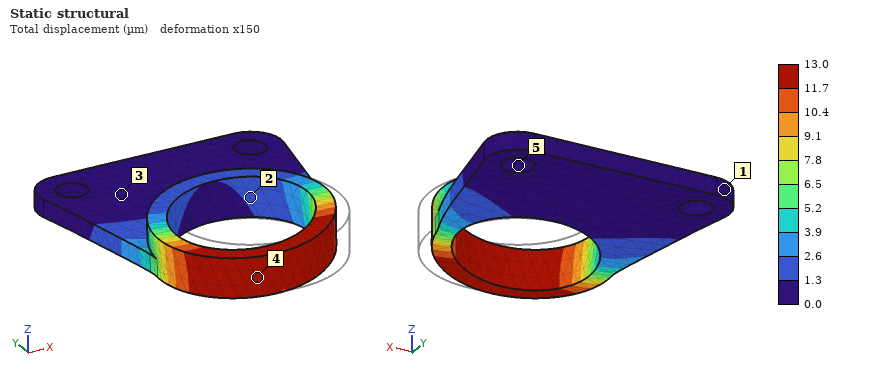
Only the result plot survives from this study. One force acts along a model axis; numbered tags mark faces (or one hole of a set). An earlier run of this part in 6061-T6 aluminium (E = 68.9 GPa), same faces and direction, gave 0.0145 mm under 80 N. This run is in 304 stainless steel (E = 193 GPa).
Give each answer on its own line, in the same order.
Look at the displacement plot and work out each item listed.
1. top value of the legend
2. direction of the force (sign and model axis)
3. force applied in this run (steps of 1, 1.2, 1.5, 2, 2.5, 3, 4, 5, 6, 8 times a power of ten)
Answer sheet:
13.0 µm
-X
200 N
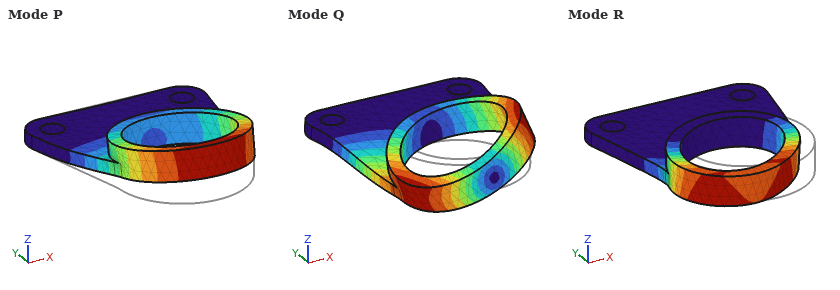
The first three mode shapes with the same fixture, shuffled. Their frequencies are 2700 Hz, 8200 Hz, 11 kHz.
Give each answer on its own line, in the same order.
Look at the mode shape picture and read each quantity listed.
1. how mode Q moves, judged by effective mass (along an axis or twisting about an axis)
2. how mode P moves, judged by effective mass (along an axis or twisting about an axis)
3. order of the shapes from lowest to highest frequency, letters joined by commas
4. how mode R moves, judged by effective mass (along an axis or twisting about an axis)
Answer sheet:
twisting about Y
along Z
P, Q, R
along X
